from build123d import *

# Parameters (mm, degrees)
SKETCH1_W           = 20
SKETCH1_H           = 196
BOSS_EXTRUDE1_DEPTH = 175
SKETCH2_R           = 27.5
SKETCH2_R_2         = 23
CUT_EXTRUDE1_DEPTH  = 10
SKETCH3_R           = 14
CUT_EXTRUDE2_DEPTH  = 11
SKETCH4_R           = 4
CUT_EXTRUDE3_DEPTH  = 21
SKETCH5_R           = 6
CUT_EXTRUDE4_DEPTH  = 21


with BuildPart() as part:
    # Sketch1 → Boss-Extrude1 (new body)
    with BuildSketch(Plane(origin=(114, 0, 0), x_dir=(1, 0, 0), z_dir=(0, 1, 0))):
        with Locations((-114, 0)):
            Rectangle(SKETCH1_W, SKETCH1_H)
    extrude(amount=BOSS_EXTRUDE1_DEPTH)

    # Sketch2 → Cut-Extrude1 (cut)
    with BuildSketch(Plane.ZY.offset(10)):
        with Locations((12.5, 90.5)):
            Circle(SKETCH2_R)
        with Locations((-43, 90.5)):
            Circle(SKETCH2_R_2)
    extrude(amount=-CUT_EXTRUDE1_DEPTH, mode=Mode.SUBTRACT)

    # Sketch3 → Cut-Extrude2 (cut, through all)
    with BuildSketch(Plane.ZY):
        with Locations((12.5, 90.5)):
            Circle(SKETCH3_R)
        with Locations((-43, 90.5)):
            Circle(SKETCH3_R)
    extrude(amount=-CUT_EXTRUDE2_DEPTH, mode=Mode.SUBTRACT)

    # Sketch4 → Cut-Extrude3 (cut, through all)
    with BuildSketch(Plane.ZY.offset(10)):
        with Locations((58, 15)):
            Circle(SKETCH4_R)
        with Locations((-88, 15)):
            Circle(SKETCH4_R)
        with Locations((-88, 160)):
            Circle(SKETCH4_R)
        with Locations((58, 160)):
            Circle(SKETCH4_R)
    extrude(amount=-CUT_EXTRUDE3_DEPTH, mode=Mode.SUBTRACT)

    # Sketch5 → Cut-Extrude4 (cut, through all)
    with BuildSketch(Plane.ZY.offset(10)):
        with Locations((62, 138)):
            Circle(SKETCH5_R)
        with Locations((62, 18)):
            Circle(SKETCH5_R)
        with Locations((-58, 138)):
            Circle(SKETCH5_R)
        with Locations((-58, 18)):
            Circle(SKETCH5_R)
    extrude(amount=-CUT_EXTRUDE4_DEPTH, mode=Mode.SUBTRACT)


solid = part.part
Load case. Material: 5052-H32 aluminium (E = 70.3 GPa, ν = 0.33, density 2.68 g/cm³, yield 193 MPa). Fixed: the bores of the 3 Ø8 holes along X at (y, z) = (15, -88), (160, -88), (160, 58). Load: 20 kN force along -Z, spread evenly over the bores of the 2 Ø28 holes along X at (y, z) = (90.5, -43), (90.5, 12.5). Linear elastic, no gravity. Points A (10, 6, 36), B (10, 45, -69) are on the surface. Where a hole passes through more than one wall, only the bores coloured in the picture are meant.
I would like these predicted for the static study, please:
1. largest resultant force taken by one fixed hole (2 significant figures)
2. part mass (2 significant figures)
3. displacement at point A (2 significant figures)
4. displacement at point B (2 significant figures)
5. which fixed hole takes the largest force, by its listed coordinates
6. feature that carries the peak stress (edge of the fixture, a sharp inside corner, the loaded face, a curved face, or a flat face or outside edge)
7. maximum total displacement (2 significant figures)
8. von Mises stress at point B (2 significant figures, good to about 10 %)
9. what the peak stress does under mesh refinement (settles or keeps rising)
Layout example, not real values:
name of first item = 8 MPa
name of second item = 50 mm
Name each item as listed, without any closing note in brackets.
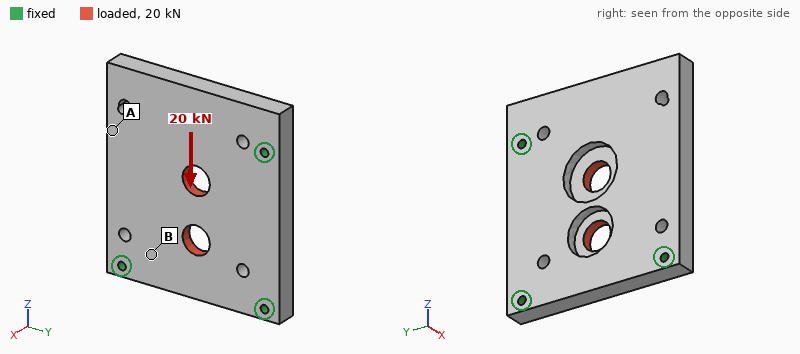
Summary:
largest resultant force taken by one fixed hole = 8.2 kN
part mass = 1.7 kg
displacement at point A = 29 µm
displacement at point B = 12 µm
which fixed hole takes the largest force, by its listed coordinates = (15, -88)
feature that carries the peak stress = edge of the fixture
maximum total displacement = 43 µm
von Mises stress at point B = 7.8 MPa
what the peak stress does under mesh refinement = keeps rising
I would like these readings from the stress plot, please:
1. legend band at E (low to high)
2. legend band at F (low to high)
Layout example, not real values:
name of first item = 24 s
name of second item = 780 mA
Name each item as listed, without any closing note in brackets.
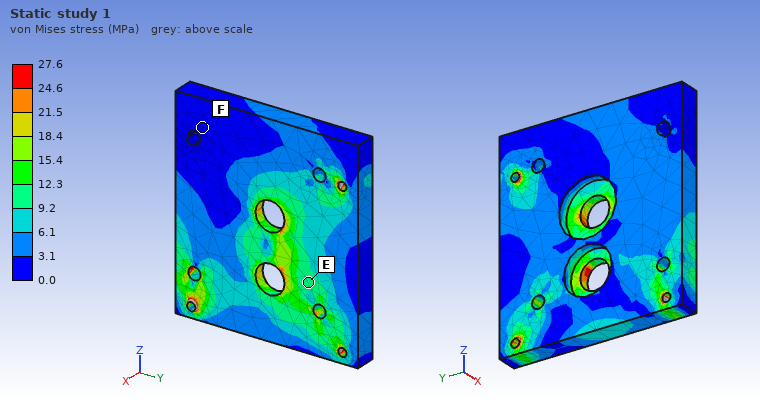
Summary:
legend band at E = 9.2 to 12.3 MPa
legend band at F = 0.0 to 3.1 MPa
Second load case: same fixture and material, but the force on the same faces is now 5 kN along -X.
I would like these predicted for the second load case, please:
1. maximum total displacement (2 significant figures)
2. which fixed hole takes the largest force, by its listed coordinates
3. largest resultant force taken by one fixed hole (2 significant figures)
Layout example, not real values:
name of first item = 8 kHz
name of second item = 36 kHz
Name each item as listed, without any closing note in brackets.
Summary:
maximum total displacement = 90 µm
which fixed hole takes the largest force, by its listed coordinates = (160, 58)
largest resultant force taken by one fixed hole = 2.2 kN
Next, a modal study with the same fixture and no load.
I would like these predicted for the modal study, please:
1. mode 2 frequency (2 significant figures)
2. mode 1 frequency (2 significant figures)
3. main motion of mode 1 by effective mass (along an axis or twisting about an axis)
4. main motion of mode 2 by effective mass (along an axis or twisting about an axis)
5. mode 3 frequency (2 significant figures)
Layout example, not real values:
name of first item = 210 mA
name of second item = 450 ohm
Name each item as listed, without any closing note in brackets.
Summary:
mode 2 frequency = 2600 Hz
mode 1 frequency = 880 Hz
main motion of mode 1 by effective mass = along X
main motion of mode 2 by effective mass = along X
mode 3 frequency = 3200 Hz
